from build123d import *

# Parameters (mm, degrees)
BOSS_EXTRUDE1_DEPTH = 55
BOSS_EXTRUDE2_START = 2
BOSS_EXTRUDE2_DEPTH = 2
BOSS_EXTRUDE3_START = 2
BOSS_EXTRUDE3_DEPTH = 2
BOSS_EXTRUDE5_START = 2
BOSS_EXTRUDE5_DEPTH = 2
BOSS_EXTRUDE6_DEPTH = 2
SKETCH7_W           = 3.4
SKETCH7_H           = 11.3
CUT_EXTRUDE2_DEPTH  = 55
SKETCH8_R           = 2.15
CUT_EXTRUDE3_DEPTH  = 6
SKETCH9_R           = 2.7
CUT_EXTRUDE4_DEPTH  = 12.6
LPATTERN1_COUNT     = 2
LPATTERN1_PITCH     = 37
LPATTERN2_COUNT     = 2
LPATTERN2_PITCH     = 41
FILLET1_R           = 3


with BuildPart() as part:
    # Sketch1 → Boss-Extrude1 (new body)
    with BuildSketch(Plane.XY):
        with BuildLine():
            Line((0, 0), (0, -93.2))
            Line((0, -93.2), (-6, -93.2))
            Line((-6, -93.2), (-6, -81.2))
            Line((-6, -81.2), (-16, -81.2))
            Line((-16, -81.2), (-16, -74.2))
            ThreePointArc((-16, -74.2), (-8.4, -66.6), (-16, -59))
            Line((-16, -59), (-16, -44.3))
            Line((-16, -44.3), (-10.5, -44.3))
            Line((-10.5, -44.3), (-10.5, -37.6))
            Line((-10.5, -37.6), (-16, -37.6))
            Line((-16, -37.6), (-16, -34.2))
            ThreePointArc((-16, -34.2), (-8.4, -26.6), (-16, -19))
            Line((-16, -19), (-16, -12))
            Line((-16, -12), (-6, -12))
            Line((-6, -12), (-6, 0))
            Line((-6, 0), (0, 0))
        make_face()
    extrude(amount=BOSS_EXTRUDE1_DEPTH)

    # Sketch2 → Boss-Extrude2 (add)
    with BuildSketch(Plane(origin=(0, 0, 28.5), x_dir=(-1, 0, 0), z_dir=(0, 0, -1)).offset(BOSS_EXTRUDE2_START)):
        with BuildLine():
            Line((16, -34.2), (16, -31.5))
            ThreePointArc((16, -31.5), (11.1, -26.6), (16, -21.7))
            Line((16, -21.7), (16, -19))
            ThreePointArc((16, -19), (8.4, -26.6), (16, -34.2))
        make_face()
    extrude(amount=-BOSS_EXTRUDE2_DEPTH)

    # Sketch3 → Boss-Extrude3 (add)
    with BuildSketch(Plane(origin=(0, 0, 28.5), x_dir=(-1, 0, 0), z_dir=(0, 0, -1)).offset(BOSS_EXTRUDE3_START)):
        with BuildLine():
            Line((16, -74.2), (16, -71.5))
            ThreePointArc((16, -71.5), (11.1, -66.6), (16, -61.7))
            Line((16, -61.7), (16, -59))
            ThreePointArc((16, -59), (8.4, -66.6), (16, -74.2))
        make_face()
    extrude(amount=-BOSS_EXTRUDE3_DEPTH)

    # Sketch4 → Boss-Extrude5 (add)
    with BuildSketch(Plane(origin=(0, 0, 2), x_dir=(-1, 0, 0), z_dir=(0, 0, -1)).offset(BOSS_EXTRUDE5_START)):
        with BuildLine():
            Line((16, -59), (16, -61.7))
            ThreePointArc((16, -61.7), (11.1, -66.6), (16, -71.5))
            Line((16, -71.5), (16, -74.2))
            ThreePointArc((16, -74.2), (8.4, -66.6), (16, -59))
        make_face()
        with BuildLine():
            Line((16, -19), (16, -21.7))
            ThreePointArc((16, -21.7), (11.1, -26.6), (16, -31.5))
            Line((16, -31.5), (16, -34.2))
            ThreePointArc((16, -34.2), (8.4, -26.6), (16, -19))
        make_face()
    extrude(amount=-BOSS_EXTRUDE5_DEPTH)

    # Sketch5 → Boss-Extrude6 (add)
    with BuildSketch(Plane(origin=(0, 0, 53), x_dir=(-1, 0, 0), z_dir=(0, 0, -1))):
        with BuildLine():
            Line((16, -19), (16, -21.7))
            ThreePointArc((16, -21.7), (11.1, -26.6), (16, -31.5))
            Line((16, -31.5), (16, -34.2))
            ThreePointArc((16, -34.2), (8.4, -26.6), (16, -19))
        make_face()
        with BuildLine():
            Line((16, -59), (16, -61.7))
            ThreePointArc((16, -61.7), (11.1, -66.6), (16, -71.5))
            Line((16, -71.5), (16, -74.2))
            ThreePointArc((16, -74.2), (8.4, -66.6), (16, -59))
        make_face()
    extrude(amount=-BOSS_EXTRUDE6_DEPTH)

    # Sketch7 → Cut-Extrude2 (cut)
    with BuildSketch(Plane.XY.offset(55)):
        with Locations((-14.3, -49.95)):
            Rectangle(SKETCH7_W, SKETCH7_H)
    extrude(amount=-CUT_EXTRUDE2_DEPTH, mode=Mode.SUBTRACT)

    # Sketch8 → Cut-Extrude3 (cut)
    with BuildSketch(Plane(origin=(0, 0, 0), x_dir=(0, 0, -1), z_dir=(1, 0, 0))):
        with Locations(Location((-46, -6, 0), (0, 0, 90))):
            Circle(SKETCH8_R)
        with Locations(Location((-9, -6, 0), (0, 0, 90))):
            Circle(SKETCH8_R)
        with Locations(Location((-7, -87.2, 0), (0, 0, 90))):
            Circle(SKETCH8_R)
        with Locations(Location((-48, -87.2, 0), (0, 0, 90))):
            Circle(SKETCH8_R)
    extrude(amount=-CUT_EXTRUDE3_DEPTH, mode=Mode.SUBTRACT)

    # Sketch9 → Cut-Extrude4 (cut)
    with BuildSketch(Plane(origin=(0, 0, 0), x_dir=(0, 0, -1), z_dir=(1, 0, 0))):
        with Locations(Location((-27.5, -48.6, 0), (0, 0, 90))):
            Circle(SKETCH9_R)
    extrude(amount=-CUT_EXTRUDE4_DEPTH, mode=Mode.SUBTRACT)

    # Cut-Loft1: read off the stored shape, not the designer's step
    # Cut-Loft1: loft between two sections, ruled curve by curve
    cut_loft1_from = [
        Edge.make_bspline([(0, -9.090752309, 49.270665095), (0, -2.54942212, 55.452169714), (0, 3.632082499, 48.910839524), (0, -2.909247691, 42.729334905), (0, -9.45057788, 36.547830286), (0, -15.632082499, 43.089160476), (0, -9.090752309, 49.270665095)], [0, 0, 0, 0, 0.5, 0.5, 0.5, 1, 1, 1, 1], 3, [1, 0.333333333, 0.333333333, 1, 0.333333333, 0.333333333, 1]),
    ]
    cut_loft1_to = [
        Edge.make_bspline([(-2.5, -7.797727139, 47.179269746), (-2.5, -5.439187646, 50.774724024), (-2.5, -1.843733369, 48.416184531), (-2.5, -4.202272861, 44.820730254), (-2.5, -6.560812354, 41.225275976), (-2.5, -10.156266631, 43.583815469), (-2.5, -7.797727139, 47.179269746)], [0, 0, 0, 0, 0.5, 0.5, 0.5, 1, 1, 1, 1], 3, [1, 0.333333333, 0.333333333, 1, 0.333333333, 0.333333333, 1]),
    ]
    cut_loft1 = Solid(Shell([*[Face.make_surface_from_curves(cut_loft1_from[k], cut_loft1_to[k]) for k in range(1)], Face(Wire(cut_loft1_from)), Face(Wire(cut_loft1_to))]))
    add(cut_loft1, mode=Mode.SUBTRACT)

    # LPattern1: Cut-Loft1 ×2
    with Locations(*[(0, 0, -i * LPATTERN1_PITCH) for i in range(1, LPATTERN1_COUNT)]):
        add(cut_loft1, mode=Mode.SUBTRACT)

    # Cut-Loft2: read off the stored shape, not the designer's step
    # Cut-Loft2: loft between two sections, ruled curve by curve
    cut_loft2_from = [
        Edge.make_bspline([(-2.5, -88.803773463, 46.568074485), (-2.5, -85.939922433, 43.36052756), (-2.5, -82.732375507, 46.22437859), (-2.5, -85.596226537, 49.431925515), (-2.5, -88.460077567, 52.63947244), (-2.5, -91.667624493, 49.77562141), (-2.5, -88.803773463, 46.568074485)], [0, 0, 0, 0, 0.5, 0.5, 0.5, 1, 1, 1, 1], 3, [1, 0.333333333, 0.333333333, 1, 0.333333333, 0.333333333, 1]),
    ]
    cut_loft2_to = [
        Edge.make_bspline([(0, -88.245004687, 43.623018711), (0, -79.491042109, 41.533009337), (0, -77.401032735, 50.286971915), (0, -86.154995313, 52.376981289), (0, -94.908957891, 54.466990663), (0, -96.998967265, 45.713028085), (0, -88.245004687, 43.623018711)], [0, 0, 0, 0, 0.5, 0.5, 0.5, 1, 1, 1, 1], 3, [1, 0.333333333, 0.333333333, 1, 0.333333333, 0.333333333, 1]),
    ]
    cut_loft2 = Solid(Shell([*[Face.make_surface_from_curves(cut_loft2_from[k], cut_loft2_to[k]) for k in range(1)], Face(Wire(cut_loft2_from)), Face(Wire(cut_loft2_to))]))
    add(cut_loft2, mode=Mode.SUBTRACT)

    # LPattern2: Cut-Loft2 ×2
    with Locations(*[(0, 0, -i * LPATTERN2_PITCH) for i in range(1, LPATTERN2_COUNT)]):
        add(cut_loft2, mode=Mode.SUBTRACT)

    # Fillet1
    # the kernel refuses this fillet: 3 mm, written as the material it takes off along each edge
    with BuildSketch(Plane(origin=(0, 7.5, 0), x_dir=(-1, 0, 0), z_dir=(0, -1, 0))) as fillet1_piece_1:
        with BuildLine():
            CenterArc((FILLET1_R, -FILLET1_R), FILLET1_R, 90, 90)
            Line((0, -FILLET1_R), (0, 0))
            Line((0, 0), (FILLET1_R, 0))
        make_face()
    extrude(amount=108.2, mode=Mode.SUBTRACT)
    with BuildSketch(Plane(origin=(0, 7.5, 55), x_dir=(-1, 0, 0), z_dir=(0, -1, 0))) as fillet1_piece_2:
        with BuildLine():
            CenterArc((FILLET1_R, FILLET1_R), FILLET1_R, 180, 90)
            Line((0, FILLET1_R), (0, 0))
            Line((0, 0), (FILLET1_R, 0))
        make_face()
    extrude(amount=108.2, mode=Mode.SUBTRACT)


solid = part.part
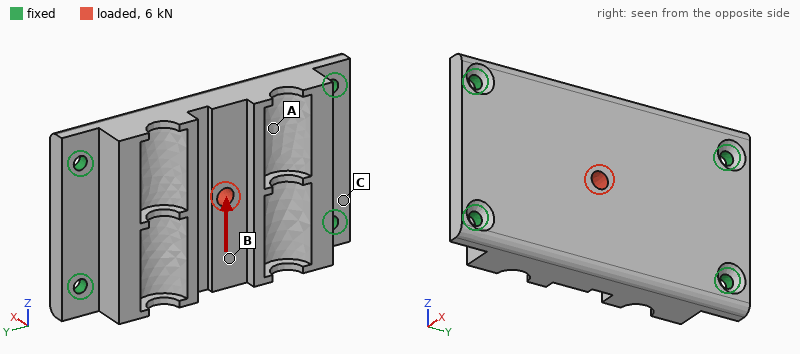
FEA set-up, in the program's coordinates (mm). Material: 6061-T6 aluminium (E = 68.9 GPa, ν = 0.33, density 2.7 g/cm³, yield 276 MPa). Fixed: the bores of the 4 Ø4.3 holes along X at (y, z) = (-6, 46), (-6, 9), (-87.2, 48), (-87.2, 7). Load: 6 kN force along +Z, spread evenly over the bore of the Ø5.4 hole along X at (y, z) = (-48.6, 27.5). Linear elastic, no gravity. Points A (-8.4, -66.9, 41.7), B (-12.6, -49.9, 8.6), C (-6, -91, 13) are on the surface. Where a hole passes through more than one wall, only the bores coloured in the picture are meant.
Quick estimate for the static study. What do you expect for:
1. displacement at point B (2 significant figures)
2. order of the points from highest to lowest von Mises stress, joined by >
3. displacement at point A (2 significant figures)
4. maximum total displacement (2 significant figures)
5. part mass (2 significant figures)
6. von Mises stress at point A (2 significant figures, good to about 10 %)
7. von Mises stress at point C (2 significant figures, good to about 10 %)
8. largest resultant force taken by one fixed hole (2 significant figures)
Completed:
18 µm
A > C > B
12 µm
20 µm
150 g
22 MPa
14 MPa
2.0 kN
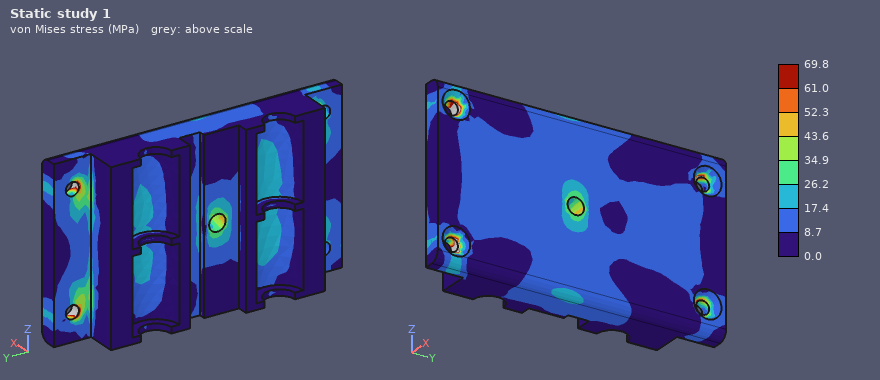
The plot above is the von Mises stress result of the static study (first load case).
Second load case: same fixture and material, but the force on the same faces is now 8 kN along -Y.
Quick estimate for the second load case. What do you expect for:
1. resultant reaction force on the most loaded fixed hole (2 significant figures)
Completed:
2.1 kN
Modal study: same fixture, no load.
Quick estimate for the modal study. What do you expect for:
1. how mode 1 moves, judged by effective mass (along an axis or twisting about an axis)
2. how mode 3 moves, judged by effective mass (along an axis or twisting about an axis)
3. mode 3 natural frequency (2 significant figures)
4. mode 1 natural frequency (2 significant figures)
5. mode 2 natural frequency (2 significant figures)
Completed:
along X
twisting about Z
11 kHz
4200 Hz
6600 Hz
